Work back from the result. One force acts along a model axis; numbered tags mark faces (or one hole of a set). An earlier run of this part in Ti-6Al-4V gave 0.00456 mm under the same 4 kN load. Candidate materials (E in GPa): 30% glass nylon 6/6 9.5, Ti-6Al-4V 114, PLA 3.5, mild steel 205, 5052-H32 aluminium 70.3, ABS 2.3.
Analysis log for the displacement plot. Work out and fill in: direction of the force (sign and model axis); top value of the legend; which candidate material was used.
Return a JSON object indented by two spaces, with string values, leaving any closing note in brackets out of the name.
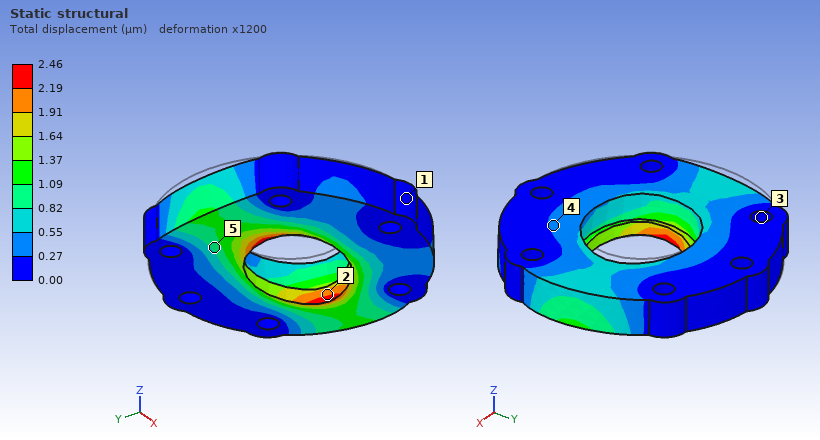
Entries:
{
  "direction of the force": "+X",
  "top value of the legend": "2.46 µm",
  "which candidate material was used": "mild steel"
}
